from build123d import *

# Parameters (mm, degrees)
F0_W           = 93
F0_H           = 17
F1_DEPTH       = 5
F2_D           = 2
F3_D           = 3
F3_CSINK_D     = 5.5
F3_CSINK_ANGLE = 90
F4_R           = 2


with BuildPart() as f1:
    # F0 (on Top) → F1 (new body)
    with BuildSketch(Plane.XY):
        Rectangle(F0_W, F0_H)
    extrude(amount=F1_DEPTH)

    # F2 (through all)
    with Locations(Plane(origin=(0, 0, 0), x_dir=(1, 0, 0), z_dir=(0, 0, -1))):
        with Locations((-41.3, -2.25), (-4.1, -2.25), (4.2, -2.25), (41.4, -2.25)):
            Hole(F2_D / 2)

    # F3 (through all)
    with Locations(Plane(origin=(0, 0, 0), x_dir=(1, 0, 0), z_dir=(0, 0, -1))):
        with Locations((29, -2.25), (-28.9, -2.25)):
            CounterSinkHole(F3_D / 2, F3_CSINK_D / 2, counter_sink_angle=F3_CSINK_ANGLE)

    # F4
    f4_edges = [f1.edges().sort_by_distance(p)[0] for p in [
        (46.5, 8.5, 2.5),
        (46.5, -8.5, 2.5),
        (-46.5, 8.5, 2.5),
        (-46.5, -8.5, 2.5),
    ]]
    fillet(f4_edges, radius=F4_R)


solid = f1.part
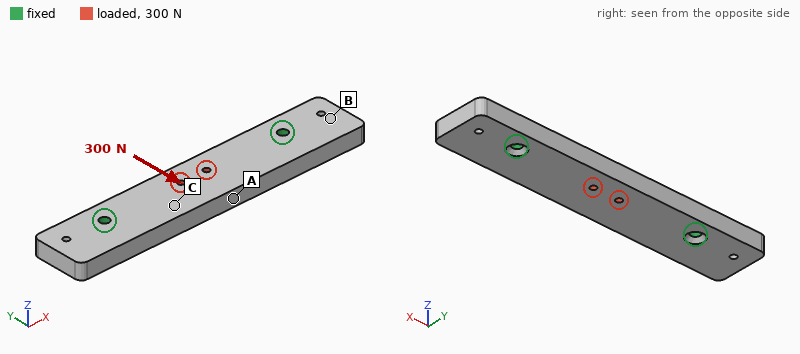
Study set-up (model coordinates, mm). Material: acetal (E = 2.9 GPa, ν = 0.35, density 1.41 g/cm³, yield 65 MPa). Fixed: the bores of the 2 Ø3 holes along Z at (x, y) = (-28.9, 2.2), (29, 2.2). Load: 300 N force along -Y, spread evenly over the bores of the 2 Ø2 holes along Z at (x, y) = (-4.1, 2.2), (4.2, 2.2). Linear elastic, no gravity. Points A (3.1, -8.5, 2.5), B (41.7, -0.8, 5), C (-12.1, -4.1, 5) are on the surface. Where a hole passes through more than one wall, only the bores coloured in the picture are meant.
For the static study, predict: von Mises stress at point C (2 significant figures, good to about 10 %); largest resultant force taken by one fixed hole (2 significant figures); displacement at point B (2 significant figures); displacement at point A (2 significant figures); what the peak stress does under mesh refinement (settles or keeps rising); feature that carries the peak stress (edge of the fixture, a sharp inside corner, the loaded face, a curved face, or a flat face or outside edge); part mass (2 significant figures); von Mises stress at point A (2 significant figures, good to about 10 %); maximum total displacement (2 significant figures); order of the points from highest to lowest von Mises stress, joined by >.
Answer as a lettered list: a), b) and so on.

a) 5.6 MPa
b) 180 N
c) 0.069 mm
d) 0.17 mm
e) keeps rising
f) edge of the fixture
g) 11 g
h) 13 MPa
i) 0.18 mm
j) A > C > B
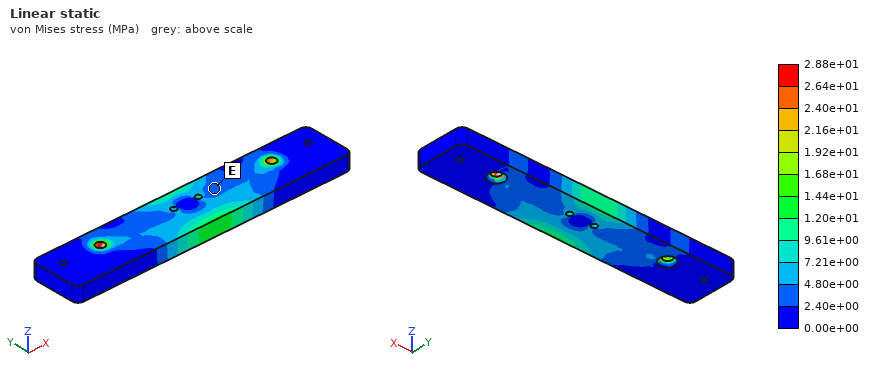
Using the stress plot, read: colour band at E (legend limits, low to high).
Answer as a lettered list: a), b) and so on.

a) 2.40e+00 to 4.80e+00 MPa
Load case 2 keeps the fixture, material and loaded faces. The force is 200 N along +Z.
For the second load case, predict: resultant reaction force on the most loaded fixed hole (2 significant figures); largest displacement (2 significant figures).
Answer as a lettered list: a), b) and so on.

a) 110 N
b) 0.56 mm
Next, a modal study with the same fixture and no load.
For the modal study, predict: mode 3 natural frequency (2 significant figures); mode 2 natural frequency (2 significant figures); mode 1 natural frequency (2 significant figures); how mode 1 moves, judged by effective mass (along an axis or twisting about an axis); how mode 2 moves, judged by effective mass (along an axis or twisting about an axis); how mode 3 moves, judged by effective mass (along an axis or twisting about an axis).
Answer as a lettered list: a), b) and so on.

a) 3000 Hz
b) 2900 Hz
c) 1800 Hz
d) along Z
e) twisting about Y
f) along Z
